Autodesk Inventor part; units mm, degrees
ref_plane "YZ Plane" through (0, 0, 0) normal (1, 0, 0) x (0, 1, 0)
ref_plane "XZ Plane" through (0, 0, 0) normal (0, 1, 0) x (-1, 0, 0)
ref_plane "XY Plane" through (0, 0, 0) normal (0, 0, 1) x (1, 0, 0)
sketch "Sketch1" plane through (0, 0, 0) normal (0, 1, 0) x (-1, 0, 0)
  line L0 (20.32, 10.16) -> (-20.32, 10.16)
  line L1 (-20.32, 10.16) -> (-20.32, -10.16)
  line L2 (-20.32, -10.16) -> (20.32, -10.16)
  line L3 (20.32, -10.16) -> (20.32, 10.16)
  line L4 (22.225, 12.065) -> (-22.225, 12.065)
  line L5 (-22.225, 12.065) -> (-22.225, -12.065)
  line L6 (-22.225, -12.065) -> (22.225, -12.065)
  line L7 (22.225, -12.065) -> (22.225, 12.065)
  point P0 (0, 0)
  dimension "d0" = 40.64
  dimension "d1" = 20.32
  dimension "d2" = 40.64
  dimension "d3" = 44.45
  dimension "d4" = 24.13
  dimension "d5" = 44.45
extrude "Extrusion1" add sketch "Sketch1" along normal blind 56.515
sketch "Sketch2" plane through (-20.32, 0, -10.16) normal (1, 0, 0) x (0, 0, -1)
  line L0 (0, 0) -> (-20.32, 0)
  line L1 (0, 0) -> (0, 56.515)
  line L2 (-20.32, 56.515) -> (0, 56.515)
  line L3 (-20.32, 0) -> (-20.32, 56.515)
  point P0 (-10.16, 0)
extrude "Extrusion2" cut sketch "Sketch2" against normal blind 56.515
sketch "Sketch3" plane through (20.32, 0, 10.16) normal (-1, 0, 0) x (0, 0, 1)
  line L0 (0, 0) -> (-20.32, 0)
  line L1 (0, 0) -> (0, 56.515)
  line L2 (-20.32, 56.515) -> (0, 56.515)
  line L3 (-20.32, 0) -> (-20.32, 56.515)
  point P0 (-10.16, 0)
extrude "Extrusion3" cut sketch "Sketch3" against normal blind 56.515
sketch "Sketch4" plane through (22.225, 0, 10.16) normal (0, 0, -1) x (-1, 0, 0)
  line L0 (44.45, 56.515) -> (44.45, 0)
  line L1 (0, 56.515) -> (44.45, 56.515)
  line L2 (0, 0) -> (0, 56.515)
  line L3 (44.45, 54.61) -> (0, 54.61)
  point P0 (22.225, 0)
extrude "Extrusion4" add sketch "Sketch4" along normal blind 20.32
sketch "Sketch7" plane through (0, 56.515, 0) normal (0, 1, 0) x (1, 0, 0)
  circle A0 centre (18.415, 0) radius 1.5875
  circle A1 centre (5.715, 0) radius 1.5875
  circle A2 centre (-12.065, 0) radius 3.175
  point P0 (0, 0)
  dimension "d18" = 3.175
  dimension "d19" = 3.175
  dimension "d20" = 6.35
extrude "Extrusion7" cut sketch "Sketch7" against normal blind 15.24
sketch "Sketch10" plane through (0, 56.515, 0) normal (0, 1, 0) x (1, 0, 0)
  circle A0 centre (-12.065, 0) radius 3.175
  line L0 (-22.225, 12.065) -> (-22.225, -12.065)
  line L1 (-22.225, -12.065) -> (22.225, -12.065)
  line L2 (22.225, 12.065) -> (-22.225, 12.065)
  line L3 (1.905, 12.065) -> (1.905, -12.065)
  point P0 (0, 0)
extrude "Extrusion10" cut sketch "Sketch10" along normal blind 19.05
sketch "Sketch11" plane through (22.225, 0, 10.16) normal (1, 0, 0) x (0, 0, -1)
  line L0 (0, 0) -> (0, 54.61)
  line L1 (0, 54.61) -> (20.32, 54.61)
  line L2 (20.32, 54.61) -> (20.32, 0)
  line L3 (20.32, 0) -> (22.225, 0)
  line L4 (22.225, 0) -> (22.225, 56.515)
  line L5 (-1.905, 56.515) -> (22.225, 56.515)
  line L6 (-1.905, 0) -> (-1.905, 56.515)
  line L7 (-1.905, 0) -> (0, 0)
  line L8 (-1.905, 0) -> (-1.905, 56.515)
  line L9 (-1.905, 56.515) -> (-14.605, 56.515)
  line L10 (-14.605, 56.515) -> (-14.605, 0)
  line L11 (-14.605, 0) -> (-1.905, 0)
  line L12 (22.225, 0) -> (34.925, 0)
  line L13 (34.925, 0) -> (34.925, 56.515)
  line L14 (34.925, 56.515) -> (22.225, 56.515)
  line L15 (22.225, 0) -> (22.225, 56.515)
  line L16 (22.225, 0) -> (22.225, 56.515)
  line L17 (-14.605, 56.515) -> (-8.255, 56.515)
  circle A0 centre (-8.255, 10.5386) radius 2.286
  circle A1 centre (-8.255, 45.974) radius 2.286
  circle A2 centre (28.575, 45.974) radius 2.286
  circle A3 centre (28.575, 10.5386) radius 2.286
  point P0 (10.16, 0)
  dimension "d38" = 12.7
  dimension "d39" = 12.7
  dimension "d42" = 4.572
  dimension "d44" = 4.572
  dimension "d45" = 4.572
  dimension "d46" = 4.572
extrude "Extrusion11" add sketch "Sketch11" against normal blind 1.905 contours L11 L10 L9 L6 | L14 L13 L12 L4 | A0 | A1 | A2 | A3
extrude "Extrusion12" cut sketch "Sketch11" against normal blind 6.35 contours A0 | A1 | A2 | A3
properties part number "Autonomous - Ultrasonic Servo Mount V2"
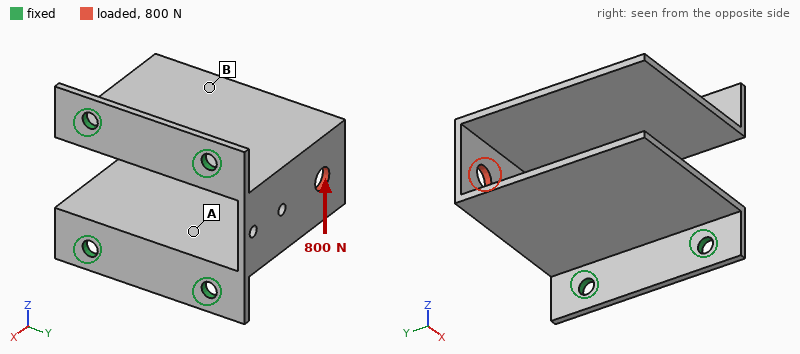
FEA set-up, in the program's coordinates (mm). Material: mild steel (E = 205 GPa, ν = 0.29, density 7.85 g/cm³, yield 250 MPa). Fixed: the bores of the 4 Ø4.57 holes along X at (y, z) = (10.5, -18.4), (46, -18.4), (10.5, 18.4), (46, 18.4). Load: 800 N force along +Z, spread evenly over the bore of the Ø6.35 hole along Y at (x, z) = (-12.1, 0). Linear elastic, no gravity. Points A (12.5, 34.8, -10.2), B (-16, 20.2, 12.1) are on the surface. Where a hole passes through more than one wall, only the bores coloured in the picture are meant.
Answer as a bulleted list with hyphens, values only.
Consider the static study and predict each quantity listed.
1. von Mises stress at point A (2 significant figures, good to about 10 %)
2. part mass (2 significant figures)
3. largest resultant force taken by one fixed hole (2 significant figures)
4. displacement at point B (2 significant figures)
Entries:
- 38 MPa
- 110 g
- 1.1 kN
- 0.083 mm
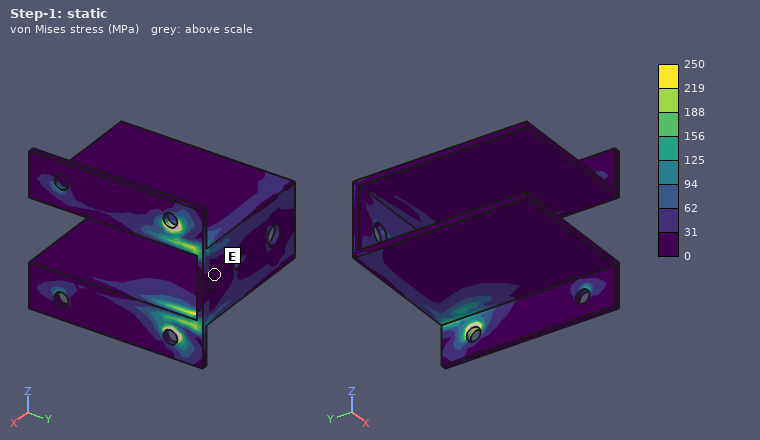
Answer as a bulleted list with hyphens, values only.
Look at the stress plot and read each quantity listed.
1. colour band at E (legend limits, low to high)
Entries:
- 0 to 31 MPa
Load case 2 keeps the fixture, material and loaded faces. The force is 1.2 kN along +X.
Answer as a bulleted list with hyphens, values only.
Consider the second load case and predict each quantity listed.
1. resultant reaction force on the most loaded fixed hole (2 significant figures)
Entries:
- 760 N
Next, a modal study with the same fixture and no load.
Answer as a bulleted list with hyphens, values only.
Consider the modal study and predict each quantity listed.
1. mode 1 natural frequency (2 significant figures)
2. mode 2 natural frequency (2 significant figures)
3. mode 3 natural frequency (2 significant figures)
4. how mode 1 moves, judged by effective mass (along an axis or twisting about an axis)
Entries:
- 1100 Hz
- 1100 Hz
- 2900 Hz
- along Z
